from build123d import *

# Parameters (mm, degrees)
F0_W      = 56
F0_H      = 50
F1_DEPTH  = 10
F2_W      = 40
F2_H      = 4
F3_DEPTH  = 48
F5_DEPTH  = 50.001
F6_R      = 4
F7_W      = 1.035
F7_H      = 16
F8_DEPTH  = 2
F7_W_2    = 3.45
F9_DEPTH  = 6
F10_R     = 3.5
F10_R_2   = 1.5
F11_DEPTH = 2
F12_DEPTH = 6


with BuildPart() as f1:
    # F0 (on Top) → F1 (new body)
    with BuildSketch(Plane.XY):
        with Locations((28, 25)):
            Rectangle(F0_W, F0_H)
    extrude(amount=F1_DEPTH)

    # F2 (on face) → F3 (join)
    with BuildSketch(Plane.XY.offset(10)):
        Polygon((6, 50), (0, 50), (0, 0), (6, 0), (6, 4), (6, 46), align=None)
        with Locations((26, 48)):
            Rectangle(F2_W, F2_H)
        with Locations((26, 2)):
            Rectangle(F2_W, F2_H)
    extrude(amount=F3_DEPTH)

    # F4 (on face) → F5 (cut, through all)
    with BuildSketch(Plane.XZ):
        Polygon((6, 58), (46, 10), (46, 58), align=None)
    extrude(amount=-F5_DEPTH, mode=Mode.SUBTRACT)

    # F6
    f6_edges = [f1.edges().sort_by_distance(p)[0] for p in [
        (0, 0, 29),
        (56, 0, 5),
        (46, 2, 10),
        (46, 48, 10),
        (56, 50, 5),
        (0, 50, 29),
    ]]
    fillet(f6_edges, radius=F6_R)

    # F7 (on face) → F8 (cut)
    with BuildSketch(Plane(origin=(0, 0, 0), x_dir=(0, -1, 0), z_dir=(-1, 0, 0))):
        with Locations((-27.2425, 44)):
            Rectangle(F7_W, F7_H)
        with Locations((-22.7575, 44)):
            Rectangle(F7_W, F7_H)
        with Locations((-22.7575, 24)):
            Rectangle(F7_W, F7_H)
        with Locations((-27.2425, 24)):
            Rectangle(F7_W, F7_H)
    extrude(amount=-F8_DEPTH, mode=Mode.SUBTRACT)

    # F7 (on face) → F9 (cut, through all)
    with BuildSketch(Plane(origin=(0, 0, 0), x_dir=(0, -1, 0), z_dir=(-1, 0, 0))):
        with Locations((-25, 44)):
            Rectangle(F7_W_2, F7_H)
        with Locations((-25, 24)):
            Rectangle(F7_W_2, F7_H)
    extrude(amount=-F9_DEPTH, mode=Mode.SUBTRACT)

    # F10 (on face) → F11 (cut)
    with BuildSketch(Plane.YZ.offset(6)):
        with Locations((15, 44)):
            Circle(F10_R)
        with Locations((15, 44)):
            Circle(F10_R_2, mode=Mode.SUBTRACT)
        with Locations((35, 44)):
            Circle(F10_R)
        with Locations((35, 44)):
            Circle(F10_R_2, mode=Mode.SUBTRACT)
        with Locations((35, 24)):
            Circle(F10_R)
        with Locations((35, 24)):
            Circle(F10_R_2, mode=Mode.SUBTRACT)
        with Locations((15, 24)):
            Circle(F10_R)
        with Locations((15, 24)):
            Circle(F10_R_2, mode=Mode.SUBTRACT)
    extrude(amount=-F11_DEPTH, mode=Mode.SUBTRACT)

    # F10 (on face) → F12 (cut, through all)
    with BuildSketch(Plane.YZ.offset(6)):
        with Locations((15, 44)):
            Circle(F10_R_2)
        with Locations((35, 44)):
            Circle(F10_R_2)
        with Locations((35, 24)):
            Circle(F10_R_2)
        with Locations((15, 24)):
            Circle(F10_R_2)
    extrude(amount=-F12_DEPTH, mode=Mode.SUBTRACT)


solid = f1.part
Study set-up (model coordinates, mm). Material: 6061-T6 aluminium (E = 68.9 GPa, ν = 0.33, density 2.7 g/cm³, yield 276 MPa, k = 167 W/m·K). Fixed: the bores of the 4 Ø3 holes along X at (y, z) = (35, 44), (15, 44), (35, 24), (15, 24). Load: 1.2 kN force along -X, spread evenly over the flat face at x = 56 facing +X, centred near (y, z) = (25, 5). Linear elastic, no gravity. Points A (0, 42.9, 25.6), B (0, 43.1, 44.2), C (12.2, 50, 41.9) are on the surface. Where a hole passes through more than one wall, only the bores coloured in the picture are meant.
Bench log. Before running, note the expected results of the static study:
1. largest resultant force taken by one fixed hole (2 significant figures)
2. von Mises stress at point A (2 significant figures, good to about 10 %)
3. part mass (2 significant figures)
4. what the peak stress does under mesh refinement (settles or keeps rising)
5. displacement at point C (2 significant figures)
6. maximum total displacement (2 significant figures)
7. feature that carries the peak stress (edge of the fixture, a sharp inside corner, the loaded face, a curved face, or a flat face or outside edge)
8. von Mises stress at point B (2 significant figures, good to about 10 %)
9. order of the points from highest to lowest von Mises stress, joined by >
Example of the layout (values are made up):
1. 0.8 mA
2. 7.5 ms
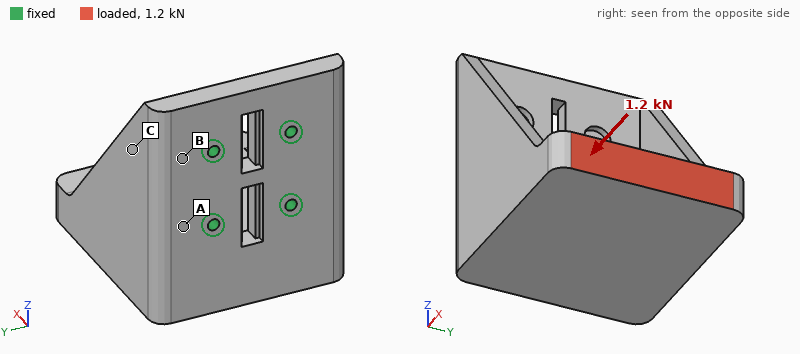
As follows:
1. 1.1 kN
2. 17 MPa
3. 130 g
4. keeps rising
5. 12 µm
6. 75 µm
7. edge of the fixture
8. 10 MPa
9. A > B > C
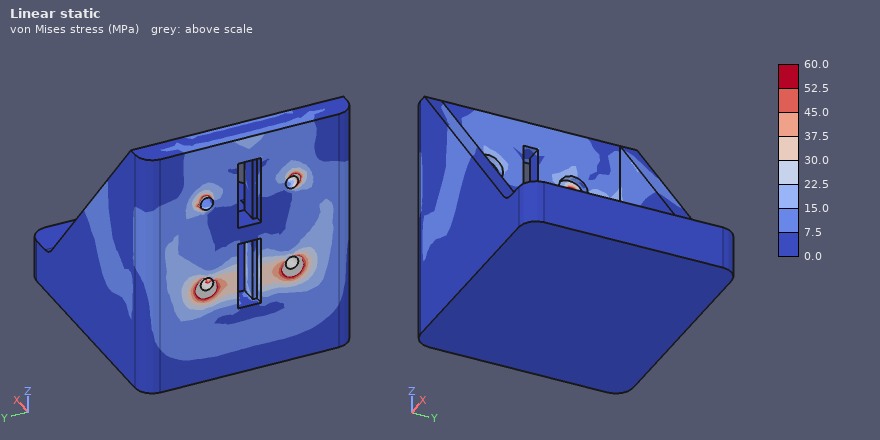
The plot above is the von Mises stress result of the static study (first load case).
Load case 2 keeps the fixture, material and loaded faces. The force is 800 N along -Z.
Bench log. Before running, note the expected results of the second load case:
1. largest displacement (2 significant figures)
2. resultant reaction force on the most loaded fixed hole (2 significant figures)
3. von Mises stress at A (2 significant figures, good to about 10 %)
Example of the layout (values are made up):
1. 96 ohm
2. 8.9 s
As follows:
1. 0.15 mm
2. 1.0 kN
3. 26 MPa
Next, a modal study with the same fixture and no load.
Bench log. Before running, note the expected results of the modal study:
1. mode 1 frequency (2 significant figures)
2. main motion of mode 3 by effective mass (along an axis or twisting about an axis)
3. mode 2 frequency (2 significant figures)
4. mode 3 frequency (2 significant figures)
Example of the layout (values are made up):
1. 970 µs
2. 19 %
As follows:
1. 2100 Hz
2. along X
3. 2100 Hz
4. 5800 Hz
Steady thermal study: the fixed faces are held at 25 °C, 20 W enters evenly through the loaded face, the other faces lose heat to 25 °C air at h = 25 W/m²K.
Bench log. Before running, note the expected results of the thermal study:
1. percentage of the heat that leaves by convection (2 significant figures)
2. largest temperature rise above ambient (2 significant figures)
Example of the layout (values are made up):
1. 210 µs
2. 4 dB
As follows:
1. 12 %
2. 16 K
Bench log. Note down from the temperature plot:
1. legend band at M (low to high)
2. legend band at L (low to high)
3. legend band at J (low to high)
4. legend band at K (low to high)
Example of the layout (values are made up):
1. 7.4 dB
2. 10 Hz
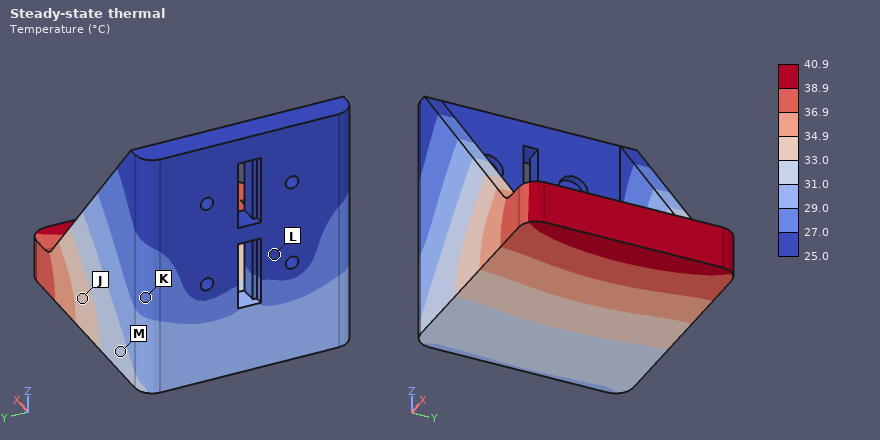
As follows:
1. 31.0 to 33.0 °C
2. 25.0 to 27.0 °C
3. 33.0 to 34.9 °C
4. 27.0 to 29.0 °C
